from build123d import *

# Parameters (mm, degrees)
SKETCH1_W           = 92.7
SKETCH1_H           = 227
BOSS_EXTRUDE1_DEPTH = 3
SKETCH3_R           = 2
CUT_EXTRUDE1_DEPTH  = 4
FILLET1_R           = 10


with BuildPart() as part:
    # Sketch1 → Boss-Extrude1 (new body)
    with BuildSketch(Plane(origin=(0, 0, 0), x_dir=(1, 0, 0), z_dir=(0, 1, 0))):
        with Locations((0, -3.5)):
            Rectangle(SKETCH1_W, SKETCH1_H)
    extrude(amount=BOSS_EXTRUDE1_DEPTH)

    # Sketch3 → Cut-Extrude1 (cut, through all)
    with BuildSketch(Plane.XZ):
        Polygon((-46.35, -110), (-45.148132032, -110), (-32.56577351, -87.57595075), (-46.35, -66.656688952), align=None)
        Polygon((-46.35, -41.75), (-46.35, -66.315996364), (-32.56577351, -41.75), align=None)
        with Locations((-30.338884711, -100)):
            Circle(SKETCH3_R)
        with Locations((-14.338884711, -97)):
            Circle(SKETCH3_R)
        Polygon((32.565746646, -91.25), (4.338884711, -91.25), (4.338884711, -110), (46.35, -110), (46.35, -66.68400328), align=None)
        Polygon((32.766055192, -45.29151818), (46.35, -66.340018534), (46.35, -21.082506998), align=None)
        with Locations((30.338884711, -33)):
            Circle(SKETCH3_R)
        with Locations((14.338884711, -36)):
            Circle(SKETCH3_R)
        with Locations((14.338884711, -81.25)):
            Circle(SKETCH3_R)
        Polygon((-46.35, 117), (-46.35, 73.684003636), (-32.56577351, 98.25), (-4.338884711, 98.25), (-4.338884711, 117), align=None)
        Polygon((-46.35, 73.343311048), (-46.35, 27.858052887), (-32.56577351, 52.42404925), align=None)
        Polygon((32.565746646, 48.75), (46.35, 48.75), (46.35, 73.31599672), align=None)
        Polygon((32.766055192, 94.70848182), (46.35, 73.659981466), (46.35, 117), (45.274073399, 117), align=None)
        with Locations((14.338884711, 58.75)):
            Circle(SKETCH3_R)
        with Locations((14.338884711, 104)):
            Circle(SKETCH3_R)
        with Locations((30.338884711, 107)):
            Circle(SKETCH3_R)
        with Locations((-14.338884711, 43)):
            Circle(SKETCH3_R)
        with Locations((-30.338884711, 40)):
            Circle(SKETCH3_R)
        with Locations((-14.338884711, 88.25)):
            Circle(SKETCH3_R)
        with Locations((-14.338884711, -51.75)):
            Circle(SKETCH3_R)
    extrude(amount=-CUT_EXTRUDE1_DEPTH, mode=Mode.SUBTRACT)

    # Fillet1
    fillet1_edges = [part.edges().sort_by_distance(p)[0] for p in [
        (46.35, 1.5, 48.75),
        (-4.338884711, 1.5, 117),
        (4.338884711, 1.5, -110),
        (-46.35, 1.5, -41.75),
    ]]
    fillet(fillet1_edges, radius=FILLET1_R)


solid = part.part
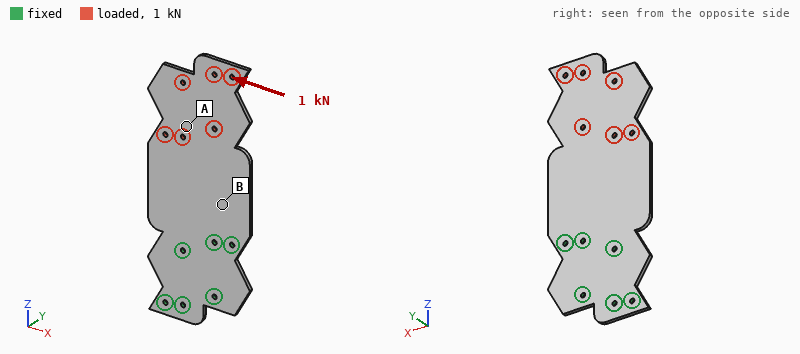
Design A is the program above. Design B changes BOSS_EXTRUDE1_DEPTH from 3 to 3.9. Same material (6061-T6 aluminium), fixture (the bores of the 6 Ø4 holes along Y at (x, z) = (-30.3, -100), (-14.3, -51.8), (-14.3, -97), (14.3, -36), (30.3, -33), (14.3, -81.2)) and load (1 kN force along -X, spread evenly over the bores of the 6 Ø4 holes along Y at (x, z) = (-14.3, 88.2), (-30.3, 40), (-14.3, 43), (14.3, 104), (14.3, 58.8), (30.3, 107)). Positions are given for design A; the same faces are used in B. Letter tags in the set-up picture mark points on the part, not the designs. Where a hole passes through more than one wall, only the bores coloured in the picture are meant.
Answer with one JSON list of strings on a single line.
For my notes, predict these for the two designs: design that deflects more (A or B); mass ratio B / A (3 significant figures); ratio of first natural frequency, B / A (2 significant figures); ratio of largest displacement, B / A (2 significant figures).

["A", "1.30", "1.3", "0.77"]
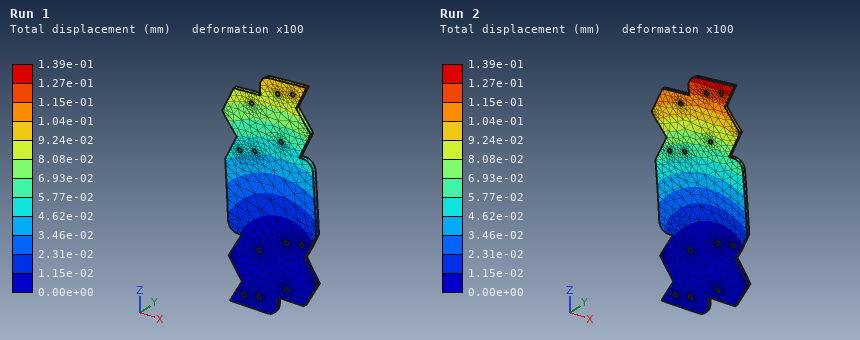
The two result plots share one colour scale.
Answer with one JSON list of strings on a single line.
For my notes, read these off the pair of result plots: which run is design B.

["Run 1"]
